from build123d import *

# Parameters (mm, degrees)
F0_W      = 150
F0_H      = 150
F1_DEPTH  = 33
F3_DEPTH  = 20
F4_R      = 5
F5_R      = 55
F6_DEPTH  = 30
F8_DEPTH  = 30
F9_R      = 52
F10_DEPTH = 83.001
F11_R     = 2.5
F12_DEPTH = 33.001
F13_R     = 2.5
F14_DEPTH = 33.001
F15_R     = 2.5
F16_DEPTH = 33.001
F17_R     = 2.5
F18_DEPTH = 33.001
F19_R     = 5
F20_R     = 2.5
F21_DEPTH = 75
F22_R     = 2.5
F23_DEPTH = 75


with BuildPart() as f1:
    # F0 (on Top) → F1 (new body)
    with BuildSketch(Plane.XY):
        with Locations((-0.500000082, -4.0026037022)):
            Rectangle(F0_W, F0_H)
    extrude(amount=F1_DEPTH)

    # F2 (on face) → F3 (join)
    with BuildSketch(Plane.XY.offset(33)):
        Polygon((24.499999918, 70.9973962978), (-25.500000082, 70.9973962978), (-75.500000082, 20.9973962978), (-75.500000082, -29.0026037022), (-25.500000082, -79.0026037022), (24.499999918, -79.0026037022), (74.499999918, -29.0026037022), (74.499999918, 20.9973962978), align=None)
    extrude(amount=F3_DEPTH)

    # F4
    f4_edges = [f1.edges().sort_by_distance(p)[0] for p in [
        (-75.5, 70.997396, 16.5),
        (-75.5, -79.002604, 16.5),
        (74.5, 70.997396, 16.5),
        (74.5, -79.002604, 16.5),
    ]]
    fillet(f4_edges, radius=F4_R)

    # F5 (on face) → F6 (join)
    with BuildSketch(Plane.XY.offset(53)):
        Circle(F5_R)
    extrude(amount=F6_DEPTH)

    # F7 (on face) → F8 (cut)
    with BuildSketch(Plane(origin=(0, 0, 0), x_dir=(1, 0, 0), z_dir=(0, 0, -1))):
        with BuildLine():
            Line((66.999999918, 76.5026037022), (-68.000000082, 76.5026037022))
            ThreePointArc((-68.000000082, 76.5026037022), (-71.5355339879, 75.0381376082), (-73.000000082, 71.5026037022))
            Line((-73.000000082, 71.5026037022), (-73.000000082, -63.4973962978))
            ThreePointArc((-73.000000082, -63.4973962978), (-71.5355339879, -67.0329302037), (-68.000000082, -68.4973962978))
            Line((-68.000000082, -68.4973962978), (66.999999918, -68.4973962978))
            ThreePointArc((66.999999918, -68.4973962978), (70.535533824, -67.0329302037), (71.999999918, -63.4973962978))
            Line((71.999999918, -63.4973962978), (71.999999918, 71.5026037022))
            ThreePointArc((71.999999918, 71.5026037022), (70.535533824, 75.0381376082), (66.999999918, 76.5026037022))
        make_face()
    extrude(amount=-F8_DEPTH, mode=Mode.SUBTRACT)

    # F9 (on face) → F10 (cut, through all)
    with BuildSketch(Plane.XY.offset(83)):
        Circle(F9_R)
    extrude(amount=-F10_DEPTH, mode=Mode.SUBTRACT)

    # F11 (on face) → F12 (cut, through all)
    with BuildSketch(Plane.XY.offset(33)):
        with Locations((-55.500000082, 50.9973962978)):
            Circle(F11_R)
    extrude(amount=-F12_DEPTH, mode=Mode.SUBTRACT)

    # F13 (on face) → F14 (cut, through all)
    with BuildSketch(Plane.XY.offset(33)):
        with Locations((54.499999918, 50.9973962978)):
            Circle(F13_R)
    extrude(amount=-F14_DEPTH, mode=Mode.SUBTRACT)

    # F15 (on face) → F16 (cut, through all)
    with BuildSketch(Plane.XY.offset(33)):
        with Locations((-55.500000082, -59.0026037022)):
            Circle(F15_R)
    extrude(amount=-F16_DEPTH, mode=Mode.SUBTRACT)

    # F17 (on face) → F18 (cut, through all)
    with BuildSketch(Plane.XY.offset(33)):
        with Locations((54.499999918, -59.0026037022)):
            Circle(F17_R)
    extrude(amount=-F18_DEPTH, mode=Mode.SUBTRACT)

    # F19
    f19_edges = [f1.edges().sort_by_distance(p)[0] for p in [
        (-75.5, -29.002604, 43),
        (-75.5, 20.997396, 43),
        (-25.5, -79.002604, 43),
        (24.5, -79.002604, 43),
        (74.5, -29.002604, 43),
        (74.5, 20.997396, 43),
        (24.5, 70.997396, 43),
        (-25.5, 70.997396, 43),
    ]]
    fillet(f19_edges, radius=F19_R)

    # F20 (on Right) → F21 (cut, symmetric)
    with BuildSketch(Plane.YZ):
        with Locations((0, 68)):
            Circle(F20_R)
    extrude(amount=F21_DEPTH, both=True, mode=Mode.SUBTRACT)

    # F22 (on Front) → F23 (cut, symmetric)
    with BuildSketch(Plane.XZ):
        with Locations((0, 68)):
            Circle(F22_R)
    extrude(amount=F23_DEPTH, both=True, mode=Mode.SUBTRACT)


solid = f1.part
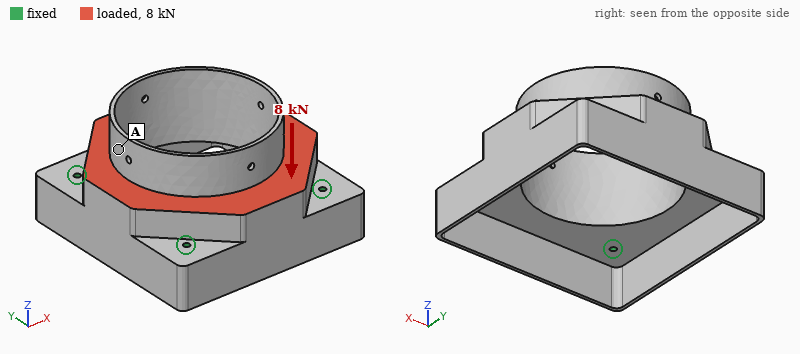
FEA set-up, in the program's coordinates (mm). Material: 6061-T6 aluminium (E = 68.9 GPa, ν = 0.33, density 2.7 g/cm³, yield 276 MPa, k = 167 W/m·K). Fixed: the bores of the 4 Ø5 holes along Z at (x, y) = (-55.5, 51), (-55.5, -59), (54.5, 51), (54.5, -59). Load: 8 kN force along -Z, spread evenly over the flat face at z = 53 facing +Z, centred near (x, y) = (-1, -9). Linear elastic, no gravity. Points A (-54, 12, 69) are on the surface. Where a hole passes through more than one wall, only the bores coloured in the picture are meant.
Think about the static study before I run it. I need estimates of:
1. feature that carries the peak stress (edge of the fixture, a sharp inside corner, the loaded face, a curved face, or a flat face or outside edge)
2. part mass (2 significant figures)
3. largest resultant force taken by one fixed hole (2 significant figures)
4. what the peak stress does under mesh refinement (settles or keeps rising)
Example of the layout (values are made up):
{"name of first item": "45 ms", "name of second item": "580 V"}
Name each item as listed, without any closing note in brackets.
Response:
{"feature that carries the peak stress": "edge of the fixture", "part mass": "800 g", "largest resultant force taken by one fixed hole": "2.4 kN", "what the peak stress does under mesh refinement": "keeps rising"}
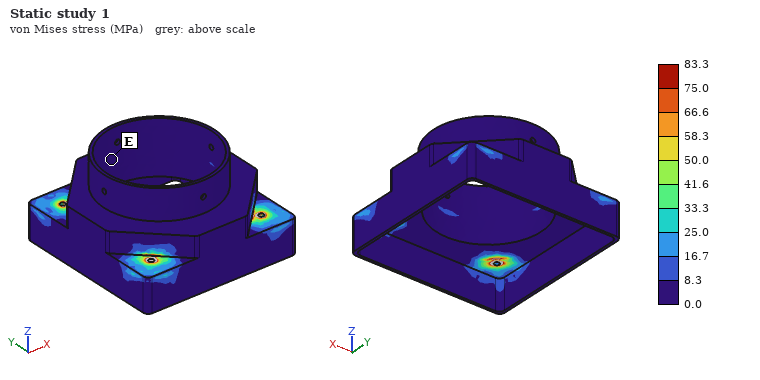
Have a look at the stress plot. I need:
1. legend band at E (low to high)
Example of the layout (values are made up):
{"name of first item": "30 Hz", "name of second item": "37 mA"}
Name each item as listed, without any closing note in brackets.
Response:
{"legend band at E": "0.0 to 8.3 MPa"}
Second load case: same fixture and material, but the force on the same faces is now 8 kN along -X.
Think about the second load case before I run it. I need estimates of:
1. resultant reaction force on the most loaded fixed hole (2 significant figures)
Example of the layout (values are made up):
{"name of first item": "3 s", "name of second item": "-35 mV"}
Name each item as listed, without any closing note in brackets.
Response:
{"resultant reaction force on the most loaded fixed hole": "2.4 kN"}
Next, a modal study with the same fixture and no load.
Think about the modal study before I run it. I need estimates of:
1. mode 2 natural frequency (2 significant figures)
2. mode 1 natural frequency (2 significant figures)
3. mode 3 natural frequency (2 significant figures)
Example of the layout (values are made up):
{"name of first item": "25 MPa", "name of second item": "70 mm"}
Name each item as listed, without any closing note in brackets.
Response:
{"mode 2 natural frequency": "2300 Hz", "mode 1 natural frequency": "2300 Hz", "mode 3 natural frequency": "2300 Hz"}
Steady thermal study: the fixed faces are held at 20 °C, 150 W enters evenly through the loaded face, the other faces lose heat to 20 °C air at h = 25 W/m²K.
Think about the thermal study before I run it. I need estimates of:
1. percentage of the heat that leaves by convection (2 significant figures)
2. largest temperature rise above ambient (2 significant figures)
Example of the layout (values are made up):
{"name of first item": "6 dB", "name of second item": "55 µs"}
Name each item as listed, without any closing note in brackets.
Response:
{"percentage of the heat that leaves by convection": "28 %", "largest temperature rise above ambient": "24 K"}
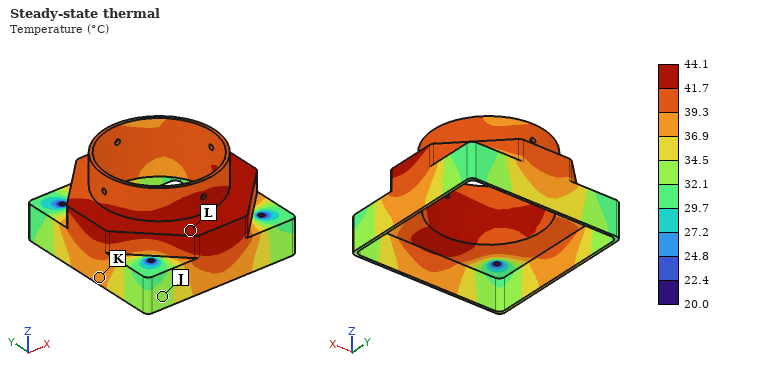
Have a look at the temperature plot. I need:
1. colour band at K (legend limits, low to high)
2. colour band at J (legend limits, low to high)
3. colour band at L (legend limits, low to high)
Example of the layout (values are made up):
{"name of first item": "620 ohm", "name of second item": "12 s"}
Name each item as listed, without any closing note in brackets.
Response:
{"colour band at K": "36.9 to 39.3 °C", "colour band at J": "32.1 to 34.5 °C", "colour band at L": "41.7 to 44.1 °C"}
